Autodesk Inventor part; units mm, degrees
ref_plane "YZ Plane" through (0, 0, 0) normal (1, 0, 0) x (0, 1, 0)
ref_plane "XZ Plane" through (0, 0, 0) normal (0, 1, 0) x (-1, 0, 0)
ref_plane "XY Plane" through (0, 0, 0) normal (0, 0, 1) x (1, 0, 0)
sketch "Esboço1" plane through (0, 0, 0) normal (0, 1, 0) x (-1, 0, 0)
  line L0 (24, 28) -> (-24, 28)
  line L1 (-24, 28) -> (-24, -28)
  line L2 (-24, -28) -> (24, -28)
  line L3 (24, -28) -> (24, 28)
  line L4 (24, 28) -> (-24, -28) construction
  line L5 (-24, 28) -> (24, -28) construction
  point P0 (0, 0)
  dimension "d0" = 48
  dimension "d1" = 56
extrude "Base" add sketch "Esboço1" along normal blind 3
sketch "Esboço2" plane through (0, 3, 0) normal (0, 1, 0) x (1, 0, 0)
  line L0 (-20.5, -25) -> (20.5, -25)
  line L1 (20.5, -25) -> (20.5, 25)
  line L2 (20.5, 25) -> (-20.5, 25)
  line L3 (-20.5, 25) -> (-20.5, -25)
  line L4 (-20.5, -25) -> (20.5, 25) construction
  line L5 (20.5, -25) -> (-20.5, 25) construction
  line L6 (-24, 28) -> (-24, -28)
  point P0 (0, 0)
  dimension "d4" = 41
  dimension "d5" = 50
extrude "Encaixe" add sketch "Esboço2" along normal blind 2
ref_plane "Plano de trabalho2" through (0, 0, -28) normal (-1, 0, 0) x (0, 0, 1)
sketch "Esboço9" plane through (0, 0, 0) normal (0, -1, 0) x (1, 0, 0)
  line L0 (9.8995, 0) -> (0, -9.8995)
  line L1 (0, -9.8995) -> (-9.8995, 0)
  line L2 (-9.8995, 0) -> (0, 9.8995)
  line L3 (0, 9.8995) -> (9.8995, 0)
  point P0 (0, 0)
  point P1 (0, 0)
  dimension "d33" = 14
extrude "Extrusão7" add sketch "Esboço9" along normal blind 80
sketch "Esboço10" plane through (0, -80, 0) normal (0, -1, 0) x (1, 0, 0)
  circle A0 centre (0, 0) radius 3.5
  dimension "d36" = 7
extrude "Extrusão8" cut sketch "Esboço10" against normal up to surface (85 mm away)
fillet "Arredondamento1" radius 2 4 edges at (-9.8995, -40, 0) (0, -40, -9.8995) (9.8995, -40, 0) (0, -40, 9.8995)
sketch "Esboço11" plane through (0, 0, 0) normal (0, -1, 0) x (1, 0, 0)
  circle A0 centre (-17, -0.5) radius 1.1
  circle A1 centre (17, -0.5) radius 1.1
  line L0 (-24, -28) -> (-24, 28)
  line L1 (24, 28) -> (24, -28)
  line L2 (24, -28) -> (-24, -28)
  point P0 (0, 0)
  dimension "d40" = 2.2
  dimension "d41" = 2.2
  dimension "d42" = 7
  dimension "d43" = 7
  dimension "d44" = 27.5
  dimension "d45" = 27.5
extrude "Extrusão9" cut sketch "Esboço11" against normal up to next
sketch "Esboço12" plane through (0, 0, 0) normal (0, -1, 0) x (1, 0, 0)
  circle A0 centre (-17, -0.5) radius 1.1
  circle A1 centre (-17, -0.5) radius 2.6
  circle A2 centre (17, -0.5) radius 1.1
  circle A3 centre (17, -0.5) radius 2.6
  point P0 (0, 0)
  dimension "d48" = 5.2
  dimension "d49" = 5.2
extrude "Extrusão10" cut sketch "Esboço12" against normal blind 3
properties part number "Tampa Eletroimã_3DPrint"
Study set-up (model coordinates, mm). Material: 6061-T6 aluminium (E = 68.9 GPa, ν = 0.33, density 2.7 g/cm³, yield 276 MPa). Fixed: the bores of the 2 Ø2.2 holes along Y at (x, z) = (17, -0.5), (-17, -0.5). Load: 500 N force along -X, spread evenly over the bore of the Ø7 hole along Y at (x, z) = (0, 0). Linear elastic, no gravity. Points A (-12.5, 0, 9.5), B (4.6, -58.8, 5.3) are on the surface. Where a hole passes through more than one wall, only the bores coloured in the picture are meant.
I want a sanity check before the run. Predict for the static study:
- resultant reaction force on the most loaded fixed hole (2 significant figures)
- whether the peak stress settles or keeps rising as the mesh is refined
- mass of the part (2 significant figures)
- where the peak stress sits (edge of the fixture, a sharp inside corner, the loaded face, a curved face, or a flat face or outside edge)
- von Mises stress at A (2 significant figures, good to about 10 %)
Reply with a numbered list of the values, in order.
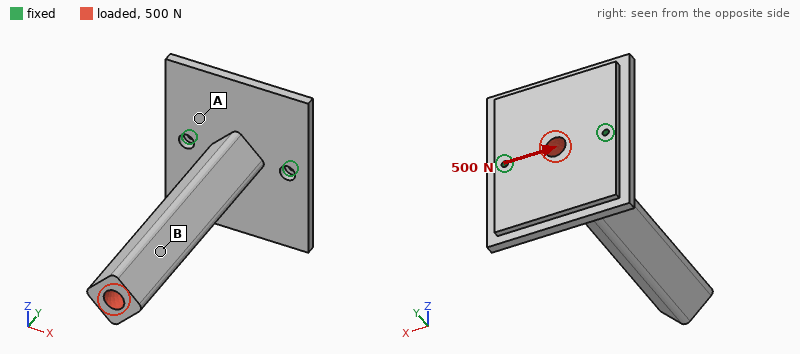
1. 690 N
2. keeps rising
3. 65 g
4. edge of the fixture
5. 16 MPa
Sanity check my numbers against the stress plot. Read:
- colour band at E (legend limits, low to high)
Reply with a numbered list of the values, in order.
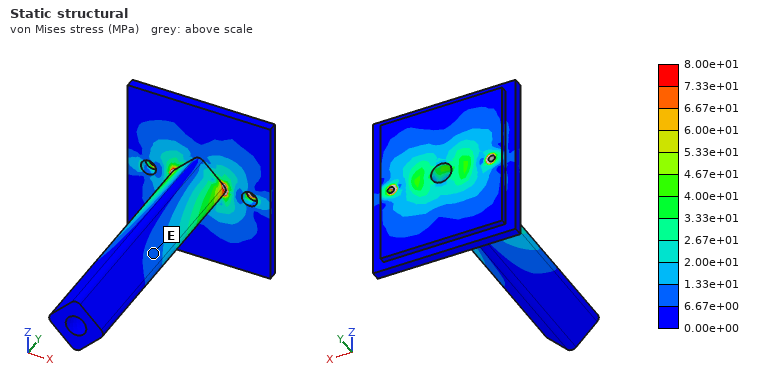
1. 6.67e+00 to 1.33e+01 MPa
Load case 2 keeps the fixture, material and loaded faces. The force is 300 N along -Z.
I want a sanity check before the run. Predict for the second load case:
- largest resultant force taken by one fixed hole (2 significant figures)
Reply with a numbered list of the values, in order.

1. 150 N
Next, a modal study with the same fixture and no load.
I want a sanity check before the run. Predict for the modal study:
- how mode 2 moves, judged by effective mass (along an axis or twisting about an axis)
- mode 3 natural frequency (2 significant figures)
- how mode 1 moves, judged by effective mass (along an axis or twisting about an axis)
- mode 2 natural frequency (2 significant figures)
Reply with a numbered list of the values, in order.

1. along X
2. 4300 Hz
3. along Z
4. 1400 Hz
